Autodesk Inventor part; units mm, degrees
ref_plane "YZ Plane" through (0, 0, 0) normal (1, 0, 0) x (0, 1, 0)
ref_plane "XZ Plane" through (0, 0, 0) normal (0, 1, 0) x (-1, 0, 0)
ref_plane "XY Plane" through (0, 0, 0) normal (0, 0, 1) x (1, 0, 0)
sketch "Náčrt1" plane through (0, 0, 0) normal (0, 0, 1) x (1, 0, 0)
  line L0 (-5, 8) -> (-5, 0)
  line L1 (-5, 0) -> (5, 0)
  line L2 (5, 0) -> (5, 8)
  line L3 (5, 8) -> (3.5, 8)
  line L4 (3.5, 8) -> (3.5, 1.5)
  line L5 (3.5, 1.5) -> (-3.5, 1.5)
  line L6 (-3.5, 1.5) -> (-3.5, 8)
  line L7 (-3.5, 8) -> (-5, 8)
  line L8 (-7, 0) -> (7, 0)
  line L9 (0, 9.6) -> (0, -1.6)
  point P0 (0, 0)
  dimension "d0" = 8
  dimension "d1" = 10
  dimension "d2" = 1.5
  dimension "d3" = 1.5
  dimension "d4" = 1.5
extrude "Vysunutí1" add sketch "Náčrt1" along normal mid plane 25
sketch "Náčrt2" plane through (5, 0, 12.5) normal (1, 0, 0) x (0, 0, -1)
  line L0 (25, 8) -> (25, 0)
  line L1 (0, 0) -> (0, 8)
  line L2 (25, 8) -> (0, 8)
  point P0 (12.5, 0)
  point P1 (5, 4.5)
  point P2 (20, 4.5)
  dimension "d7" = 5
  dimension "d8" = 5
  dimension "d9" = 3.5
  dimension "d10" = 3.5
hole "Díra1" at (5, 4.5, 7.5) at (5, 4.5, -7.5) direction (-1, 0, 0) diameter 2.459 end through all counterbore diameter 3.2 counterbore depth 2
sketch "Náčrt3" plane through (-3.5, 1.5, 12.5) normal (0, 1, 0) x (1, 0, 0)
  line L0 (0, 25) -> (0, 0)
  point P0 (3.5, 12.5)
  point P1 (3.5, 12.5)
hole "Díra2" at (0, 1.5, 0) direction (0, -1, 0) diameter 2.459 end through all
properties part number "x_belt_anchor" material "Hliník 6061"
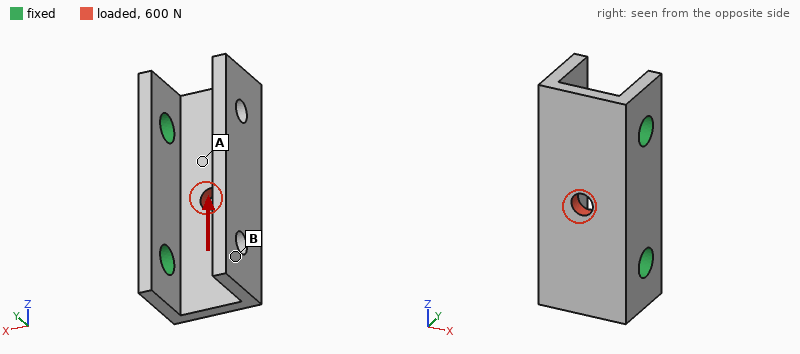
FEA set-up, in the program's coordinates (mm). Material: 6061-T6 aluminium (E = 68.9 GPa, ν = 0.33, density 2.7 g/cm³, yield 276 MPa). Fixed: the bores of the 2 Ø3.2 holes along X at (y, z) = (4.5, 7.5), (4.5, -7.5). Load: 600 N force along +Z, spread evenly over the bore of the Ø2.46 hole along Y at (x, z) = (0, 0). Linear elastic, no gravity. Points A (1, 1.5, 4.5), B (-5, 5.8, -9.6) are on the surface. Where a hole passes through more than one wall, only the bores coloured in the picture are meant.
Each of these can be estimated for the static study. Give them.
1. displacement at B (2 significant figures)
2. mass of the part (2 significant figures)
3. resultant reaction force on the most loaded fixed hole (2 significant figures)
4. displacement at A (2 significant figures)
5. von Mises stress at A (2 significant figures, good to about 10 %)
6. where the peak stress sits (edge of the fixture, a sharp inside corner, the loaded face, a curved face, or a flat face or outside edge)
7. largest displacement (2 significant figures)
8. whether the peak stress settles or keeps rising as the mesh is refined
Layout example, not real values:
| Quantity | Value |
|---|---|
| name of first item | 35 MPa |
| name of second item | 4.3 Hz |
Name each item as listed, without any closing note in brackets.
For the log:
| Quantity | Value |
|---|---|
| displacement at B | 23 µm |
| mass of the part | 2.2 g |
| resultant reaction force on the most loaded fixed hole | 350 N |
| displacement at A | 8.5 µm |
| von Mises stress at A | 47 MPa |
| where the peak stress sits | edge of the fixture |
| largest displacement | 27 µm |
| whether the peak stress settles or keeps rising as the mesh is refined | keeps rising |
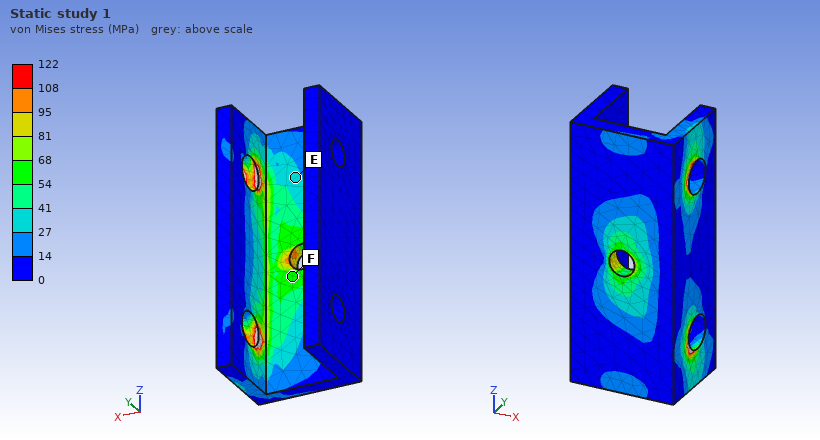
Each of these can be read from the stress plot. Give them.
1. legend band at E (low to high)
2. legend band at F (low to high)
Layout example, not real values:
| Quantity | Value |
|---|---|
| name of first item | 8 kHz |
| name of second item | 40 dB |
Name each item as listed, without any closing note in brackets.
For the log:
| Quantity | Value |
|---|---|
| legend band at E | 27 to 41 MPa |
| legend band at F | 54 to 68 MPa |
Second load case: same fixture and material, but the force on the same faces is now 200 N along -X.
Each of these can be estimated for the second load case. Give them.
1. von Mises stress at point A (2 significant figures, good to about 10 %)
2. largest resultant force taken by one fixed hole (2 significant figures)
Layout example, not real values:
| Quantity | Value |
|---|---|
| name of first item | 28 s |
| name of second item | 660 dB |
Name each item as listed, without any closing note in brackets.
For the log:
| Quantity | Value |
|---|---|
| von Mises stress at point A | 15 MPa |
| largest resultant force taken by one fixed hole | 110 N |
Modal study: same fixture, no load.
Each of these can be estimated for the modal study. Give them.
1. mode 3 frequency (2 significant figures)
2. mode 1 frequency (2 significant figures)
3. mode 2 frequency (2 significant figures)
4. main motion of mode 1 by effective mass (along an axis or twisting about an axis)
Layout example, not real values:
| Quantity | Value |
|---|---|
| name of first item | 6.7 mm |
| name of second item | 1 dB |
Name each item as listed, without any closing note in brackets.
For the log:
| Quantity | Value |
|---|---|
| mode 3 frequency | 15 kHz |
| mode 1 frequency | 5300 Hz |
| mode 2 frequency | 8600 Hz |
| main motion of mode 1 by effective mass | along Y |
